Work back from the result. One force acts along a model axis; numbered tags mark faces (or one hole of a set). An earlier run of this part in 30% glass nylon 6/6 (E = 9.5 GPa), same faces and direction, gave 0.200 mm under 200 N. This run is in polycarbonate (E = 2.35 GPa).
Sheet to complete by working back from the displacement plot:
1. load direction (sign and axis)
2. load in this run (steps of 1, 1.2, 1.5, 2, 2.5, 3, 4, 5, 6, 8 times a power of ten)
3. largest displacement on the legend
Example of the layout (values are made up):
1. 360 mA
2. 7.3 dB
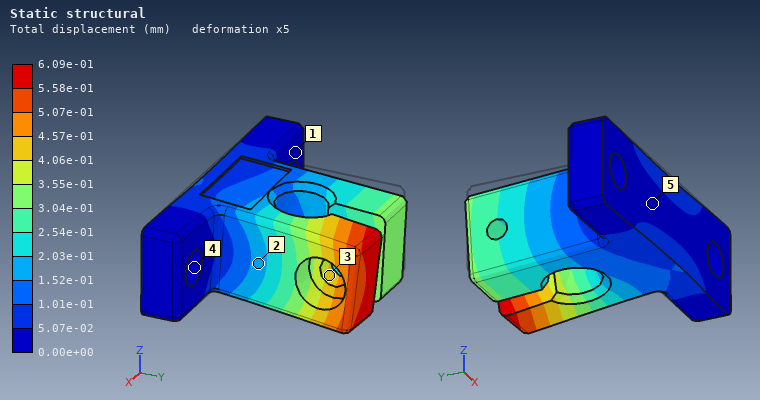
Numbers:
1. -Z
2. 150 N
3. 6.09e-01 mm
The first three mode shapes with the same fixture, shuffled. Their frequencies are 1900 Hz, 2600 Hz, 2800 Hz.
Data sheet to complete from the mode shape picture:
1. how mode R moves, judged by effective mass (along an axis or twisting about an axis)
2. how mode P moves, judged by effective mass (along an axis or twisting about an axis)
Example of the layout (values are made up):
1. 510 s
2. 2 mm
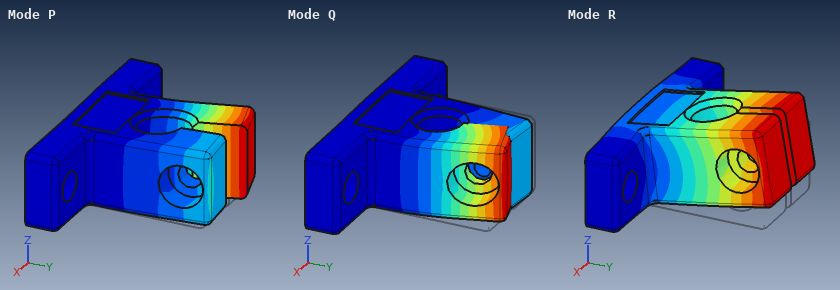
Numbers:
1. along Z
2. along X
